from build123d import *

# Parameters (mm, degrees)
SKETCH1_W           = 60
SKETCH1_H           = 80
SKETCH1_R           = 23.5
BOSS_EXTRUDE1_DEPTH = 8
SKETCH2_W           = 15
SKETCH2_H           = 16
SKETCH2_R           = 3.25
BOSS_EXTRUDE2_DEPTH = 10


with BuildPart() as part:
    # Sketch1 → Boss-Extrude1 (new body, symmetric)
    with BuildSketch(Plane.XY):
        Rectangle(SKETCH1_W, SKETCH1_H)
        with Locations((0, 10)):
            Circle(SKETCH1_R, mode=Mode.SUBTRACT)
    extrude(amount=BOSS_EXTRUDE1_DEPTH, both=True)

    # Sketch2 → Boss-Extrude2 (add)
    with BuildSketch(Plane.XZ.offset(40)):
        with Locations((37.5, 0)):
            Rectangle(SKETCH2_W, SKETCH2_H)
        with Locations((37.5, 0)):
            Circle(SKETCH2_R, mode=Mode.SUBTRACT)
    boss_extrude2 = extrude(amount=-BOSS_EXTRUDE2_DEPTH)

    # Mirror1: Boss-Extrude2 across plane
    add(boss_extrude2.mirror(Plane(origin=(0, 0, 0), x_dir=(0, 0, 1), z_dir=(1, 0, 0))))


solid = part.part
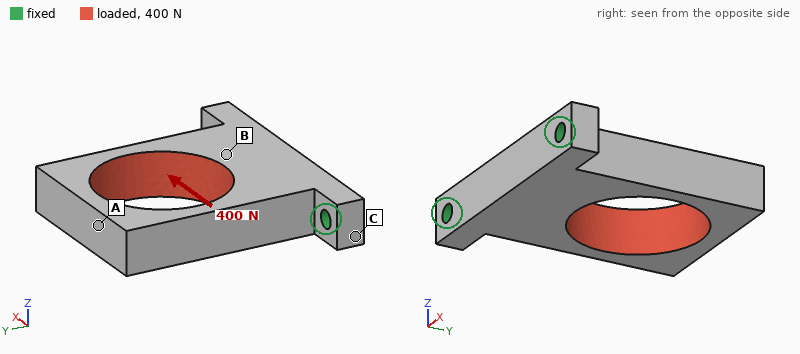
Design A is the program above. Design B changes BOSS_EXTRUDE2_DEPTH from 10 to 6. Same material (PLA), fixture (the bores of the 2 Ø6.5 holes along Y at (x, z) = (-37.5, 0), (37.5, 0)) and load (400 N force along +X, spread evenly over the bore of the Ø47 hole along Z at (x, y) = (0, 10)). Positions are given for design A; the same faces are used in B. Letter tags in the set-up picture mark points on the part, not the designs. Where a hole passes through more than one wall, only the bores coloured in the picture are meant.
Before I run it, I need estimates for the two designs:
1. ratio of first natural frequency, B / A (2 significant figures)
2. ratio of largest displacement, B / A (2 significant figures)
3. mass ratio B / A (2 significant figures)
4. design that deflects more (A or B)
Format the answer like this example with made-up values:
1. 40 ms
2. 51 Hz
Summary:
1. 0.68
2. 1.2
3. 0.97
4. B
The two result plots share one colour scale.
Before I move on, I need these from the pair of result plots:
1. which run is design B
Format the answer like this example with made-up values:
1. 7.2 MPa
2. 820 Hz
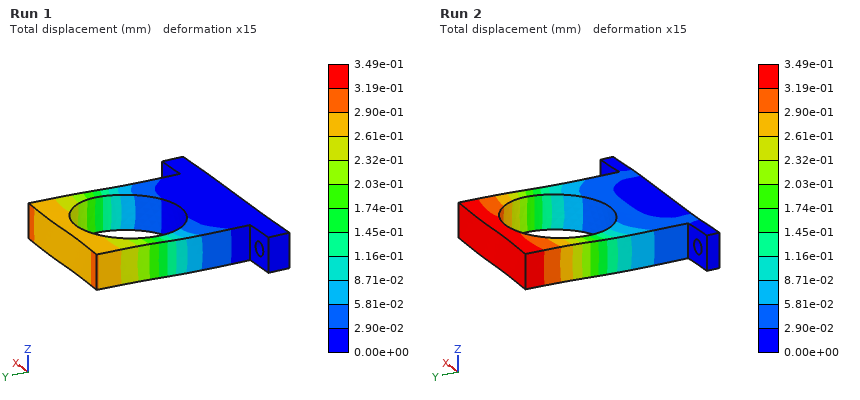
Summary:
1. Run 2
